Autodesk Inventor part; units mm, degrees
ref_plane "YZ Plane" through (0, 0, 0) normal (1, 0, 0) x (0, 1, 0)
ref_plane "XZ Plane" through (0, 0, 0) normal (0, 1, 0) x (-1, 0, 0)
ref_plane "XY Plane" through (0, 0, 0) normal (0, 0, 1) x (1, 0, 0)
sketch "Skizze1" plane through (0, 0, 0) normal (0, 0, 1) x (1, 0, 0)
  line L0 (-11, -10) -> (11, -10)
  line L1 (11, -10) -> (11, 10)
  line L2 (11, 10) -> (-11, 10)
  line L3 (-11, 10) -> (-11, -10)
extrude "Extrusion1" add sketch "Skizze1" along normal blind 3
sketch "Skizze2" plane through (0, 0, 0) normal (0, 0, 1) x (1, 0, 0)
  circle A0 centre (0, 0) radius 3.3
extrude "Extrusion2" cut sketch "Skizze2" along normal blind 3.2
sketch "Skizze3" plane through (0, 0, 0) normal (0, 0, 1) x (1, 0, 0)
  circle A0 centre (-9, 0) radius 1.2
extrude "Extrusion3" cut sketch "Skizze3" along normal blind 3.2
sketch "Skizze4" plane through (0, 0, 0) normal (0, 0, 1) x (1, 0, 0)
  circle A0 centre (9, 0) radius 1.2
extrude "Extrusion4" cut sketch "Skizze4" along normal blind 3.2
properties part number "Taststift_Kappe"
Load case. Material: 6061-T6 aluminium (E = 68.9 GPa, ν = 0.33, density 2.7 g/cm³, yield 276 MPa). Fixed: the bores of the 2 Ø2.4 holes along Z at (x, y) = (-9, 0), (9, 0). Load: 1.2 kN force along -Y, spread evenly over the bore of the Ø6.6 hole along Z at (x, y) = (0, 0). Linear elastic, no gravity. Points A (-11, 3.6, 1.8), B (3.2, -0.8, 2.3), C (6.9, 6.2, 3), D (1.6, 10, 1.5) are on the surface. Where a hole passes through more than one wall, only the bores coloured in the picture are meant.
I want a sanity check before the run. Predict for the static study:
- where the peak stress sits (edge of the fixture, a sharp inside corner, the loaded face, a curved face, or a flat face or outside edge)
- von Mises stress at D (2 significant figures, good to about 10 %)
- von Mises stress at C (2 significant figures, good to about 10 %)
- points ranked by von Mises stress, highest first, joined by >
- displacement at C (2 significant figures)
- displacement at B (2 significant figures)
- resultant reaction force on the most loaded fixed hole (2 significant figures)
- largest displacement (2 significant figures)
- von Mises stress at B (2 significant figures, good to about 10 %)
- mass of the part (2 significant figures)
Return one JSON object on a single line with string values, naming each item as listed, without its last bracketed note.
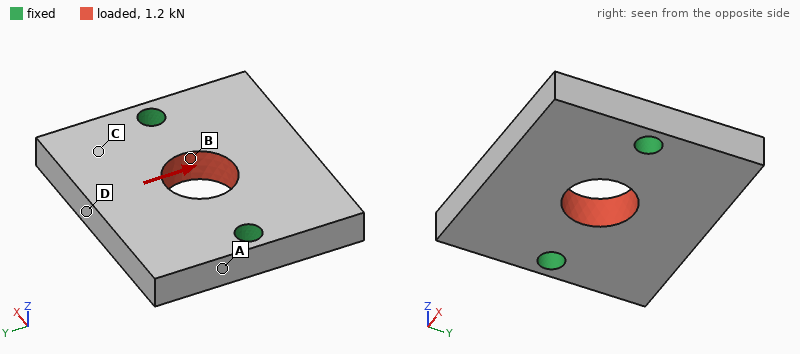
{"where the peak stress sits": "edge of the fixture", "von Mises stress at D": "25 MPa", "von Mises stress at C": "14 MPa", "points ranked by von Mises stress, highest first, joined by >": "B > D > C > A", "displacement at C": "2.0 µm", "displacement at B": "4.1 µm", "resultant reaction force on the most loaded fixed hole": "600 N", "largest displacement": "4.9 µm", "von Mises stress at B": "34 MPa", "mass of the part": "3.2 g"}
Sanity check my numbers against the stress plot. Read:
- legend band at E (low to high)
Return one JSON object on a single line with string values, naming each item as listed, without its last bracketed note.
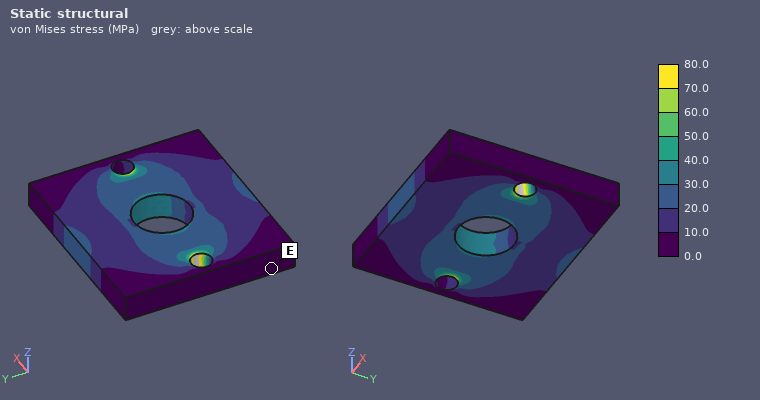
{"legend band at E": "0.0 to 10.0 MPa"}
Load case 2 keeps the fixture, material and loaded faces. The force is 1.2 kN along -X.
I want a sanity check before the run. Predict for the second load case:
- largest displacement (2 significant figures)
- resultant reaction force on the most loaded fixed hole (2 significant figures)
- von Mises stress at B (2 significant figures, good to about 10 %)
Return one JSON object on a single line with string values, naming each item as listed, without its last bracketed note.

{"largest displacement": "3.4 µm", "resultant reaction force on the most loaded fixed hole": "600 N", "von Mises stress at B": "25 MPa"}
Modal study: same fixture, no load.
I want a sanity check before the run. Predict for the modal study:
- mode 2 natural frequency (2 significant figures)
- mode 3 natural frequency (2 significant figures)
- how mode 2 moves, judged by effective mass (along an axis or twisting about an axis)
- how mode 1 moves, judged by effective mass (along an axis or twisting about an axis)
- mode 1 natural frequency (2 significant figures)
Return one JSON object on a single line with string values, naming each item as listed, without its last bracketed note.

{"mode 2 natural frequency": "21 kHz", "mode 3 natural frequency": "32 kHz", "how mode 2 moves, judged by effective mass": "along Z", "how mode 1 moves, judged by effective mass": "twisting about X", "mode 1 natural frequency": "17 kHz"}
